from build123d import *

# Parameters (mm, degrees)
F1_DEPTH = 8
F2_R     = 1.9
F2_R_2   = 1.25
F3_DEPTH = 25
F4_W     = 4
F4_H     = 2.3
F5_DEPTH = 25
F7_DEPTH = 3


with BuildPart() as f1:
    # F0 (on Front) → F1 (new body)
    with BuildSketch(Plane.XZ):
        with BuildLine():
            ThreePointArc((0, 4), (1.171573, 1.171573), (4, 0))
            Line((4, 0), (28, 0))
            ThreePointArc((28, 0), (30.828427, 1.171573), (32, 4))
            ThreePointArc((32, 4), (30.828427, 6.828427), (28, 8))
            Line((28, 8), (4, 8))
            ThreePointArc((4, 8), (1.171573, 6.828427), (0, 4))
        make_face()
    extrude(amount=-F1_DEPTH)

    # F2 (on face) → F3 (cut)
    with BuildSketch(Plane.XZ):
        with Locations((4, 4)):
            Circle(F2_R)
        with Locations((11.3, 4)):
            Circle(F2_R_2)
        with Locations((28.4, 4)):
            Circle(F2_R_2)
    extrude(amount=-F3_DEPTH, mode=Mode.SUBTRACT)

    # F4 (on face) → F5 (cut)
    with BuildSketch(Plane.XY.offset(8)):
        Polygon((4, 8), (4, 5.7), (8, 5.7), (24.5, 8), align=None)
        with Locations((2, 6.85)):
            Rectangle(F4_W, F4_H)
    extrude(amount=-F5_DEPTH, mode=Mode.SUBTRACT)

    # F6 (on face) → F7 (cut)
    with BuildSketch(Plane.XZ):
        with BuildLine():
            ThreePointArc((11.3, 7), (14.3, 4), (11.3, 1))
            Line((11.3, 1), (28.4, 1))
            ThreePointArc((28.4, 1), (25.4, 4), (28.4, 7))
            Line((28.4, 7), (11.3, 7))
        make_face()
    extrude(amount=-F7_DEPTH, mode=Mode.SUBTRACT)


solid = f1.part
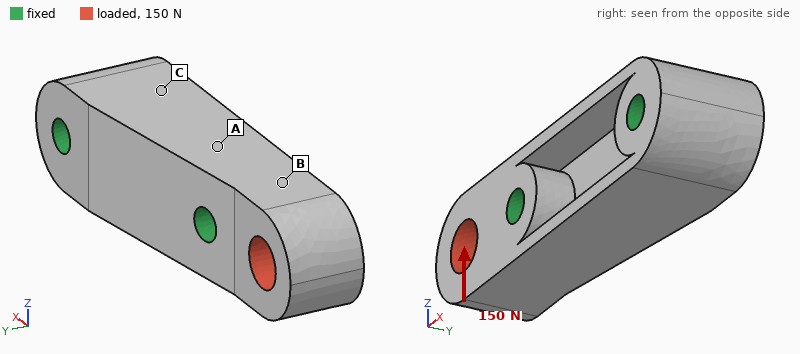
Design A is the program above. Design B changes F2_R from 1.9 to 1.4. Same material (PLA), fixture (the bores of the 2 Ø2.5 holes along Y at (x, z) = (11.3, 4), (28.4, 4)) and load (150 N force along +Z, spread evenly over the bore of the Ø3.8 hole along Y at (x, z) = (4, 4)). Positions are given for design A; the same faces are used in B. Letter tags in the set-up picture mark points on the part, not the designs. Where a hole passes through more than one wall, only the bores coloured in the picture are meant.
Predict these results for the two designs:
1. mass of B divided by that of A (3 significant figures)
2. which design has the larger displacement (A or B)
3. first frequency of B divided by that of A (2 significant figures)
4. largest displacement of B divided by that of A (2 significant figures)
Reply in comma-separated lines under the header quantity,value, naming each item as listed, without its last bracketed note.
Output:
quantity,value
mass of B divided by that of A,1.02
which design has the larger displacement,A
first frequency of B divided by that of A,1.00
largest displacement of B divided by that of A,0.89
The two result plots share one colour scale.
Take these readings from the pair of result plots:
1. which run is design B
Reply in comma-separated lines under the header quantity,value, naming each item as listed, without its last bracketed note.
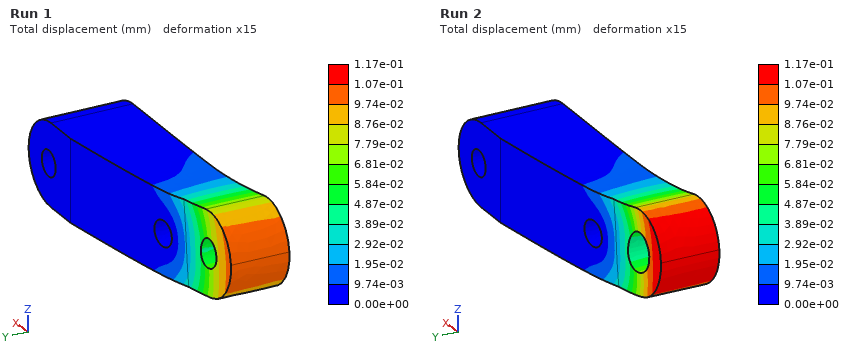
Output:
quantity,value
which run is design B,Run 1
